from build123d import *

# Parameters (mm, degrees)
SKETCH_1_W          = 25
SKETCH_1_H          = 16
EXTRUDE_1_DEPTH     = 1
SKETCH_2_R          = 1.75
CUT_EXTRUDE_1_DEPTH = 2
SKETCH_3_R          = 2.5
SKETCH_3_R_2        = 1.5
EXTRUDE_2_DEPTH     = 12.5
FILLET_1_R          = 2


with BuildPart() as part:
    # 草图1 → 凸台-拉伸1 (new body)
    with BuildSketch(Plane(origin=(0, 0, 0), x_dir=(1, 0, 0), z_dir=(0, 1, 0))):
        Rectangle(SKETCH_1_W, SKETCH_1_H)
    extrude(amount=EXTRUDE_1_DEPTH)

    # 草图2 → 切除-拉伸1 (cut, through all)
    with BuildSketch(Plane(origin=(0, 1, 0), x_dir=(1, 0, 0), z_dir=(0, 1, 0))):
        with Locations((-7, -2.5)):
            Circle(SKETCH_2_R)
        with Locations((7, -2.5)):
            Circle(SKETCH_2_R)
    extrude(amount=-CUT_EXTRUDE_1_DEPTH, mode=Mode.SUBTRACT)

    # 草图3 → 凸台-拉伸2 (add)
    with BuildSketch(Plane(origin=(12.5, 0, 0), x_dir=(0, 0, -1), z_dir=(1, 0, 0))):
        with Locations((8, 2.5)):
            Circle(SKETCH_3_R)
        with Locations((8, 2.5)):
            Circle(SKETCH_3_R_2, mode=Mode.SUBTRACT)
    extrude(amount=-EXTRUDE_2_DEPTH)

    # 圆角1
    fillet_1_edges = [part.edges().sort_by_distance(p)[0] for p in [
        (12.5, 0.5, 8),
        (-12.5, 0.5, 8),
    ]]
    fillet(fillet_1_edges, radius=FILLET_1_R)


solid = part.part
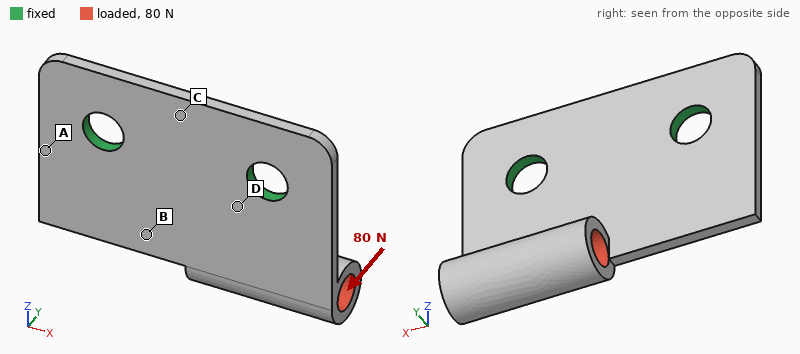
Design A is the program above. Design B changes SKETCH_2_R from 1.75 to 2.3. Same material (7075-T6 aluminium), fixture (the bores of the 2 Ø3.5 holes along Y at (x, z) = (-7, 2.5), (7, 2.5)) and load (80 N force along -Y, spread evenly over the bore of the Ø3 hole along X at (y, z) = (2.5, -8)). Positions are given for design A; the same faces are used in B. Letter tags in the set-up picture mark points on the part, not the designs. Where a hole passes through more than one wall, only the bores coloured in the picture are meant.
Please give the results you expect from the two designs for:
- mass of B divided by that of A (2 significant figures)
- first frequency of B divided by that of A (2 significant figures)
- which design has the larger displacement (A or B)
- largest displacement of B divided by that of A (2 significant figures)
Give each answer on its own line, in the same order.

0.97
1.1
A
0.84
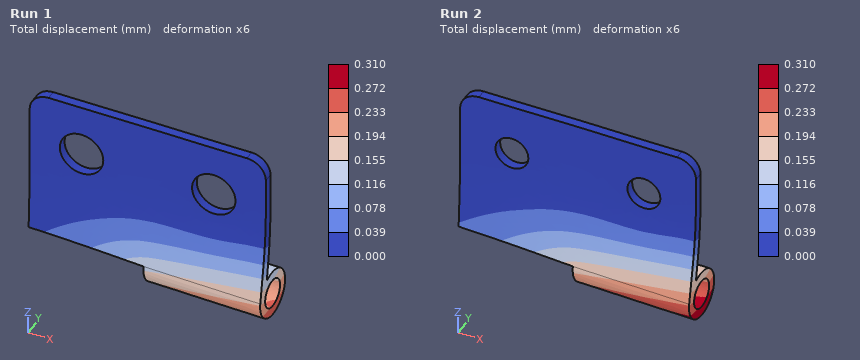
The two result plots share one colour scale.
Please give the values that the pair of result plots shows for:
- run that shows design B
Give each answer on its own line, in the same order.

Run 1
